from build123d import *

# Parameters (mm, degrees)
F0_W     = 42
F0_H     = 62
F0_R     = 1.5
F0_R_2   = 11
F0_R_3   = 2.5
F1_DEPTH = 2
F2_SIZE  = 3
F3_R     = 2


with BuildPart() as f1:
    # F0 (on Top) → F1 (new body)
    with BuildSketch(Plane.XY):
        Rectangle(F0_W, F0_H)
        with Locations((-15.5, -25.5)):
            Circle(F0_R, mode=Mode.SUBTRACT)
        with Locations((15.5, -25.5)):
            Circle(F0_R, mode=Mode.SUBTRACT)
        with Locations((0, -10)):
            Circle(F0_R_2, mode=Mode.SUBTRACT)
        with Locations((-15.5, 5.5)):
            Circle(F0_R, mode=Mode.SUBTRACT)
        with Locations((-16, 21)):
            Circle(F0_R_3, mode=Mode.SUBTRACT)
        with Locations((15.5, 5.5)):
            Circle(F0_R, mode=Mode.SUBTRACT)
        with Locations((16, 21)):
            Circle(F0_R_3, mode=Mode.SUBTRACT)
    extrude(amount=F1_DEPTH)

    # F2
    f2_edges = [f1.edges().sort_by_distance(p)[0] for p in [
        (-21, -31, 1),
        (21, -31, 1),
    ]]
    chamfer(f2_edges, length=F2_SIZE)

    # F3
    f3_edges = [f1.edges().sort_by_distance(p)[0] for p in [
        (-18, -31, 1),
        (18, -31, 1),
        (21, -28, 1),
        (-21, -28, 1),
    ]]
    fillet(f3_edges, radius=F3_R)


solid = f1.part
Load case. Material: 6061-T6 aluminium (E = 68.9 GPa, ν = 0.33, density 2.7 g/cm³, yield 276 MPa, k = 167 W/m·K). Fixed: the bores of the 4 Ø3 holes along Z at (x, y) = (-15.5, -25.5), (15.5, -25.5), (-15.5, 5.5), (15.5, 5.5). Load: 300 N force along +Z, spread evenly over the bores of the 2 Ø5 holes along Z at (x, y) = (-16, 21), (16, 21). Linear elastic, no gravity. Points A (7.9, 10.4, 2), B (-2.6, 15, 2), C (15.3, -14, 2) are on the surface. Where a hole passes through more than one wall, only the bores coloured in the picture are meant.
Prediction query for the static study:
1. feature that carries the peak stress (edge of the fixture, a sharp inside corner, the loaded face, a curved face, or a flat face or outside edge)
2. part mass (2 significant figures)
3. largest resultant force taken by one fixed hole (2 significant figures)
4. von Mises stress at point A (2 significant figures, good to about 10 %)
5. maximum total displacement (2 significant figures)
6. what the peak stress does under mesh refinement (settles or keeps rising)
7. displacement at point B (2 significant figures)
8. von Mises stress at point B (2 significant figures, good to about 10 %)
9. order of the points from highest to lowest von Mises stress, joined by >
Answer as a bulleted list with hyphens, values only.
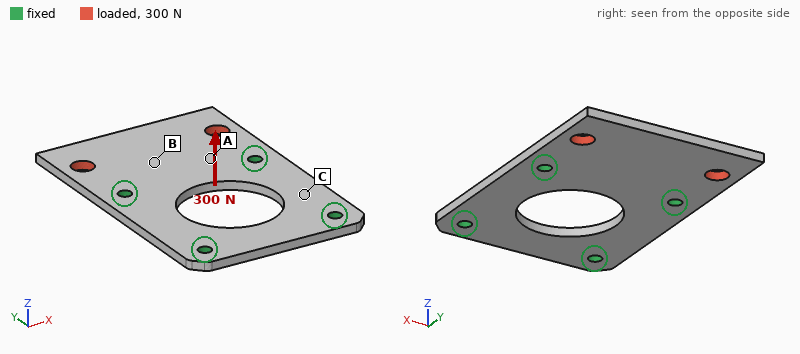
- edge of the fixture
- 12 g
- 160 N
- 83 MPa
- 0.44 mm
- keeps rising
- 0.11 mm
- 49 MPa
- A > B > C
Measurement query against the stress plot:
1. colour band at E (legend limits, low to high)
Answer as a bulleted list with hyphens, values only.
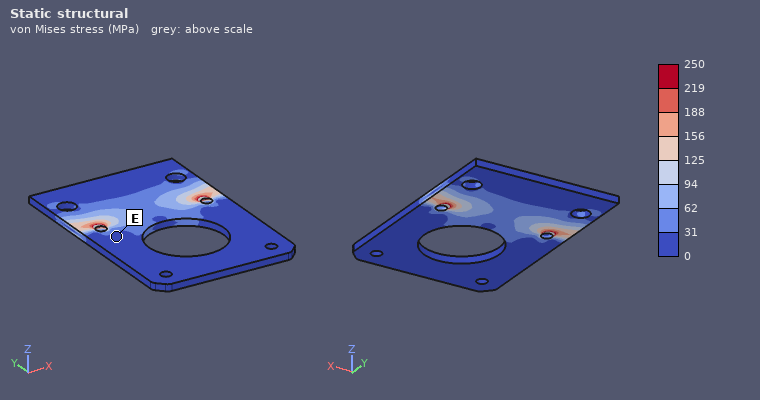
- 0 to 31 MPa
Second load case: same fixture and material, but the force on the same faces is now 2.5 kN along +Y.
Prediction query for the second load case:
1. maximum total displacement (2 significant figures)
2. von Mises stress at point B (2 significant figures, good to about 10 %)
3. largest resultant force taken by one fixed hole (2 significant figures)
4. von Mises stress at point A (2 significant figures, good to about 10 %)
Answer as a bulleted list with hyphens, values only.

- 17 µm
- 10.0 MPa
- 1.2 kN
- 15 MPa
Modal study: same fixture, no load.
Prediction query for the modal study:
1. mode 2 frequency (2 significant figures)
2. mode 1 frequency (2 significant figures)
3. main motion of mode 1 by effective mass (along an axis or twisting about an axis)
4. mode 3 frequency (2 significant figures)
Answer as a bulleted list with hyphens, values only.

- 4500 Hz
- 2300 Hz
- along Z
- 8500 Hz
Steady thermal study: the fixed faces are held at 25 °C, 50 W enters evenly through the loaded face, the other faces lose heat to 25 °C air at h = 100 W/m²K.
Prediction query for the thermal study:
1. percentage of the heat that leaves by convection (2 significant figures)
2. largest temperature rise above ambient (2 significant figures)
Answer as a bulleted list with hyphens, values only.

- 21 %
- 76 K
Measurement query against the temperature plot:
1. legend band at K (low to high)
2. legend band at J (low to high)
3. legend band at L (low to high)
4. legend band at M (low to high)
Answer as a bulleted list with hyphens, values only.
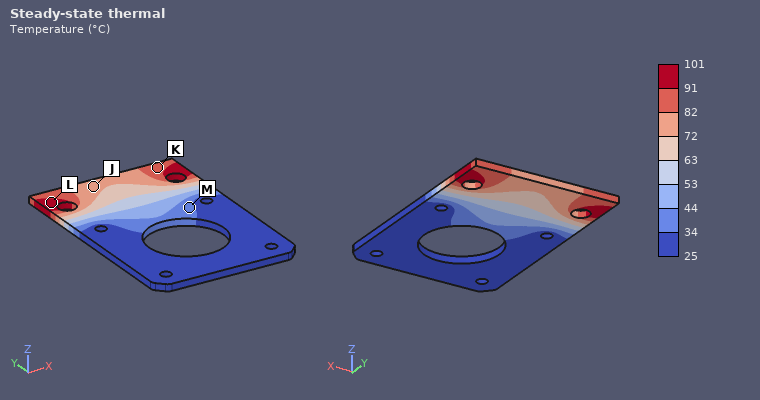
- 82 to 91 °C
- 72 to 82 °C
- 91 to 101 °C
- 34 to 44 °C
